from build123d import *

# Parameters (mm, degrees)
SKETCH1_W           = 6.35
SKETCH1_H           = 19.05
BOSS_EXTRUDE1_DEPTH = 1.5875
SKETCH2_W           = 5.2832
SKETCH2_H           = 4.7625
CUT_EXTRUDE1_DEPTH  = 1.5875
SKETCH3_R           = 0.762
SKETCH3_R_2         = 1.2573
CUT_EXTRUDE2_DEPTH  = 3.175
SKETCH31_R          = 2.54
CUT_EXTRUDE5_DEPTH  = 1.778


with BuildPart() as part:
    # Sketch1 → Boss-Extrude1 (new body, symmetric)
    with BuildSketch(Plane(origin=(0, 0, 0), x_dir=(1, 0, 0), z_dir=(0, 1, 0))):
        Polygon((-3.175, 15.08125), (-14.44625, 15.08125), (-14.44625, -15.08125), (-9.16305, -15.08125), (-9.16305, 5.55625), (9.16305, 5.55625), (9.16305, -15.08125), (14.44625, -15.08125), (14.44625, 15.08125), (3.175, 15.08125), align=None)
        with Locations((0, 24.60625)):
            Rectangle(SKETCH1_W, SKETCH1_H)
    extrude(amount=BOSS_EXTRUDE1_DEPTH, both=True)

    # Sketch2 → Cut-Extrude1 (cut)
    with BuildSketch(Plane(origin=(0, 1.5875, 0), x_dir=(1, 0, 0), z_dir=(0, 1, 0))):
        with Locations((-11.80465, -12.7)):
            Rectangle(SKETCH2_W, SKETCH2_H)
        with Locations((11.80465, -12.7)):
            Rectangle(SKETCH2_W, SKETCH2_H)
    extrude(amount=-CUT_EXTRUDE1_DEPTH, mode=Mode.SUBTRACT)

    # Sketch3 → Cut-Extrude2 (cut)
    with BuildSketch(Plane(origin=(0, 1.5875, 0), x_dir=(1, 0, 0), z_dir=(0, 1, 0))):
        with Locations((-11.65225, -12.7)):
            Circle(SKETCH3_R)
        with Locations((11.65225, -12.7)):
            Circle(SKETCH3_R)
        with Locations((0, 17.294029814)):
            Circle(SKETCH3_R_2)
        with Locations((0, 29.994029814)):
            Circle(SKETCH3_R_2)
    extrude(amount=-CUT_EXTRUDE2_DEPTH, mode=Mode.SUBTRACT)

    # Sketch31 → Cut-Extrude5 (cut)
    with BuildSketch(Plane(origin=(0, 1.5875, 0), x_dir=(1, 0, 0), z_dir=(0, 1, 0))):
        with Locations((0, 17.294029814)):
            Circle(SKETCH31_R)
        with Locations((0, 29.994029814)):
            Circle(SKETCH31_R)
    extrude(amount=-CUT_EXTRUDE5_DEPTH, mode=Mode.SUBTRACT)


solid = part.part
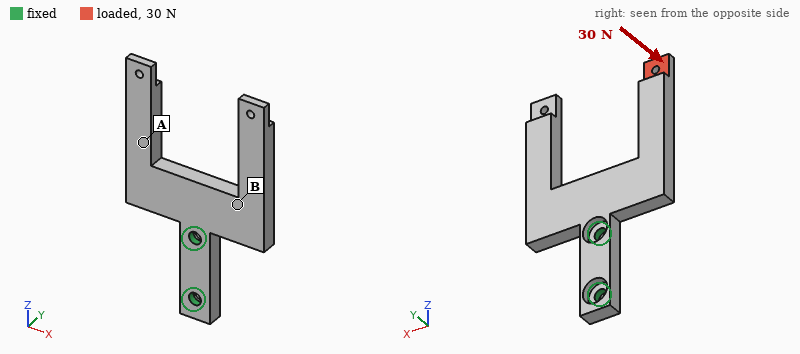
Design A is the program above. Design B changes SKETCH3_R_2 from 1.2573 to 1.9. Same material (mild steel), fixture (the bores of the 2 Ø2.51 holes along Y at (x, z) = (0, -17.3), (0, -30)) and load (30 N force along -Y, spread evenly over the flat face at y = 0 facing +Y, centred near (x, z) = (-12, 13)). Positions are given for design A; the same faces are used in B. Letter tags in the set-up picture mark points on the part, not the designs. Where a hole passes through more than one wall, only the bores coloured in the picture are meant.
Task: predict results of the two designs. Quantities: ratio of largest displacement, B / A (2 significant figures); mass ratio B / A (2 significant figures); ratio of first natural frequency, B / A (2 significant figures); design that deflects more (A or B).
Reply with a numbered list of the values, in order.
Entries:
1. 0.86
2. 0.99
3. 1.1
4. A
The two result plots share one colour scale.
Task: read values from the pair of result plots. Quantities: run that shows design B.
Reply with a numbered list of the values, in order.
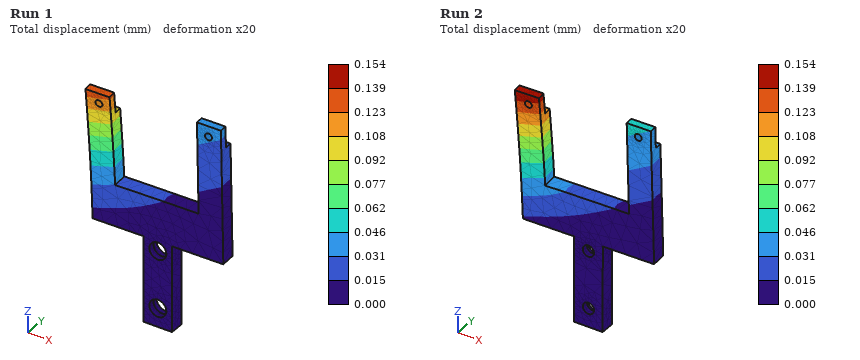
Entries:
1. Run 1
